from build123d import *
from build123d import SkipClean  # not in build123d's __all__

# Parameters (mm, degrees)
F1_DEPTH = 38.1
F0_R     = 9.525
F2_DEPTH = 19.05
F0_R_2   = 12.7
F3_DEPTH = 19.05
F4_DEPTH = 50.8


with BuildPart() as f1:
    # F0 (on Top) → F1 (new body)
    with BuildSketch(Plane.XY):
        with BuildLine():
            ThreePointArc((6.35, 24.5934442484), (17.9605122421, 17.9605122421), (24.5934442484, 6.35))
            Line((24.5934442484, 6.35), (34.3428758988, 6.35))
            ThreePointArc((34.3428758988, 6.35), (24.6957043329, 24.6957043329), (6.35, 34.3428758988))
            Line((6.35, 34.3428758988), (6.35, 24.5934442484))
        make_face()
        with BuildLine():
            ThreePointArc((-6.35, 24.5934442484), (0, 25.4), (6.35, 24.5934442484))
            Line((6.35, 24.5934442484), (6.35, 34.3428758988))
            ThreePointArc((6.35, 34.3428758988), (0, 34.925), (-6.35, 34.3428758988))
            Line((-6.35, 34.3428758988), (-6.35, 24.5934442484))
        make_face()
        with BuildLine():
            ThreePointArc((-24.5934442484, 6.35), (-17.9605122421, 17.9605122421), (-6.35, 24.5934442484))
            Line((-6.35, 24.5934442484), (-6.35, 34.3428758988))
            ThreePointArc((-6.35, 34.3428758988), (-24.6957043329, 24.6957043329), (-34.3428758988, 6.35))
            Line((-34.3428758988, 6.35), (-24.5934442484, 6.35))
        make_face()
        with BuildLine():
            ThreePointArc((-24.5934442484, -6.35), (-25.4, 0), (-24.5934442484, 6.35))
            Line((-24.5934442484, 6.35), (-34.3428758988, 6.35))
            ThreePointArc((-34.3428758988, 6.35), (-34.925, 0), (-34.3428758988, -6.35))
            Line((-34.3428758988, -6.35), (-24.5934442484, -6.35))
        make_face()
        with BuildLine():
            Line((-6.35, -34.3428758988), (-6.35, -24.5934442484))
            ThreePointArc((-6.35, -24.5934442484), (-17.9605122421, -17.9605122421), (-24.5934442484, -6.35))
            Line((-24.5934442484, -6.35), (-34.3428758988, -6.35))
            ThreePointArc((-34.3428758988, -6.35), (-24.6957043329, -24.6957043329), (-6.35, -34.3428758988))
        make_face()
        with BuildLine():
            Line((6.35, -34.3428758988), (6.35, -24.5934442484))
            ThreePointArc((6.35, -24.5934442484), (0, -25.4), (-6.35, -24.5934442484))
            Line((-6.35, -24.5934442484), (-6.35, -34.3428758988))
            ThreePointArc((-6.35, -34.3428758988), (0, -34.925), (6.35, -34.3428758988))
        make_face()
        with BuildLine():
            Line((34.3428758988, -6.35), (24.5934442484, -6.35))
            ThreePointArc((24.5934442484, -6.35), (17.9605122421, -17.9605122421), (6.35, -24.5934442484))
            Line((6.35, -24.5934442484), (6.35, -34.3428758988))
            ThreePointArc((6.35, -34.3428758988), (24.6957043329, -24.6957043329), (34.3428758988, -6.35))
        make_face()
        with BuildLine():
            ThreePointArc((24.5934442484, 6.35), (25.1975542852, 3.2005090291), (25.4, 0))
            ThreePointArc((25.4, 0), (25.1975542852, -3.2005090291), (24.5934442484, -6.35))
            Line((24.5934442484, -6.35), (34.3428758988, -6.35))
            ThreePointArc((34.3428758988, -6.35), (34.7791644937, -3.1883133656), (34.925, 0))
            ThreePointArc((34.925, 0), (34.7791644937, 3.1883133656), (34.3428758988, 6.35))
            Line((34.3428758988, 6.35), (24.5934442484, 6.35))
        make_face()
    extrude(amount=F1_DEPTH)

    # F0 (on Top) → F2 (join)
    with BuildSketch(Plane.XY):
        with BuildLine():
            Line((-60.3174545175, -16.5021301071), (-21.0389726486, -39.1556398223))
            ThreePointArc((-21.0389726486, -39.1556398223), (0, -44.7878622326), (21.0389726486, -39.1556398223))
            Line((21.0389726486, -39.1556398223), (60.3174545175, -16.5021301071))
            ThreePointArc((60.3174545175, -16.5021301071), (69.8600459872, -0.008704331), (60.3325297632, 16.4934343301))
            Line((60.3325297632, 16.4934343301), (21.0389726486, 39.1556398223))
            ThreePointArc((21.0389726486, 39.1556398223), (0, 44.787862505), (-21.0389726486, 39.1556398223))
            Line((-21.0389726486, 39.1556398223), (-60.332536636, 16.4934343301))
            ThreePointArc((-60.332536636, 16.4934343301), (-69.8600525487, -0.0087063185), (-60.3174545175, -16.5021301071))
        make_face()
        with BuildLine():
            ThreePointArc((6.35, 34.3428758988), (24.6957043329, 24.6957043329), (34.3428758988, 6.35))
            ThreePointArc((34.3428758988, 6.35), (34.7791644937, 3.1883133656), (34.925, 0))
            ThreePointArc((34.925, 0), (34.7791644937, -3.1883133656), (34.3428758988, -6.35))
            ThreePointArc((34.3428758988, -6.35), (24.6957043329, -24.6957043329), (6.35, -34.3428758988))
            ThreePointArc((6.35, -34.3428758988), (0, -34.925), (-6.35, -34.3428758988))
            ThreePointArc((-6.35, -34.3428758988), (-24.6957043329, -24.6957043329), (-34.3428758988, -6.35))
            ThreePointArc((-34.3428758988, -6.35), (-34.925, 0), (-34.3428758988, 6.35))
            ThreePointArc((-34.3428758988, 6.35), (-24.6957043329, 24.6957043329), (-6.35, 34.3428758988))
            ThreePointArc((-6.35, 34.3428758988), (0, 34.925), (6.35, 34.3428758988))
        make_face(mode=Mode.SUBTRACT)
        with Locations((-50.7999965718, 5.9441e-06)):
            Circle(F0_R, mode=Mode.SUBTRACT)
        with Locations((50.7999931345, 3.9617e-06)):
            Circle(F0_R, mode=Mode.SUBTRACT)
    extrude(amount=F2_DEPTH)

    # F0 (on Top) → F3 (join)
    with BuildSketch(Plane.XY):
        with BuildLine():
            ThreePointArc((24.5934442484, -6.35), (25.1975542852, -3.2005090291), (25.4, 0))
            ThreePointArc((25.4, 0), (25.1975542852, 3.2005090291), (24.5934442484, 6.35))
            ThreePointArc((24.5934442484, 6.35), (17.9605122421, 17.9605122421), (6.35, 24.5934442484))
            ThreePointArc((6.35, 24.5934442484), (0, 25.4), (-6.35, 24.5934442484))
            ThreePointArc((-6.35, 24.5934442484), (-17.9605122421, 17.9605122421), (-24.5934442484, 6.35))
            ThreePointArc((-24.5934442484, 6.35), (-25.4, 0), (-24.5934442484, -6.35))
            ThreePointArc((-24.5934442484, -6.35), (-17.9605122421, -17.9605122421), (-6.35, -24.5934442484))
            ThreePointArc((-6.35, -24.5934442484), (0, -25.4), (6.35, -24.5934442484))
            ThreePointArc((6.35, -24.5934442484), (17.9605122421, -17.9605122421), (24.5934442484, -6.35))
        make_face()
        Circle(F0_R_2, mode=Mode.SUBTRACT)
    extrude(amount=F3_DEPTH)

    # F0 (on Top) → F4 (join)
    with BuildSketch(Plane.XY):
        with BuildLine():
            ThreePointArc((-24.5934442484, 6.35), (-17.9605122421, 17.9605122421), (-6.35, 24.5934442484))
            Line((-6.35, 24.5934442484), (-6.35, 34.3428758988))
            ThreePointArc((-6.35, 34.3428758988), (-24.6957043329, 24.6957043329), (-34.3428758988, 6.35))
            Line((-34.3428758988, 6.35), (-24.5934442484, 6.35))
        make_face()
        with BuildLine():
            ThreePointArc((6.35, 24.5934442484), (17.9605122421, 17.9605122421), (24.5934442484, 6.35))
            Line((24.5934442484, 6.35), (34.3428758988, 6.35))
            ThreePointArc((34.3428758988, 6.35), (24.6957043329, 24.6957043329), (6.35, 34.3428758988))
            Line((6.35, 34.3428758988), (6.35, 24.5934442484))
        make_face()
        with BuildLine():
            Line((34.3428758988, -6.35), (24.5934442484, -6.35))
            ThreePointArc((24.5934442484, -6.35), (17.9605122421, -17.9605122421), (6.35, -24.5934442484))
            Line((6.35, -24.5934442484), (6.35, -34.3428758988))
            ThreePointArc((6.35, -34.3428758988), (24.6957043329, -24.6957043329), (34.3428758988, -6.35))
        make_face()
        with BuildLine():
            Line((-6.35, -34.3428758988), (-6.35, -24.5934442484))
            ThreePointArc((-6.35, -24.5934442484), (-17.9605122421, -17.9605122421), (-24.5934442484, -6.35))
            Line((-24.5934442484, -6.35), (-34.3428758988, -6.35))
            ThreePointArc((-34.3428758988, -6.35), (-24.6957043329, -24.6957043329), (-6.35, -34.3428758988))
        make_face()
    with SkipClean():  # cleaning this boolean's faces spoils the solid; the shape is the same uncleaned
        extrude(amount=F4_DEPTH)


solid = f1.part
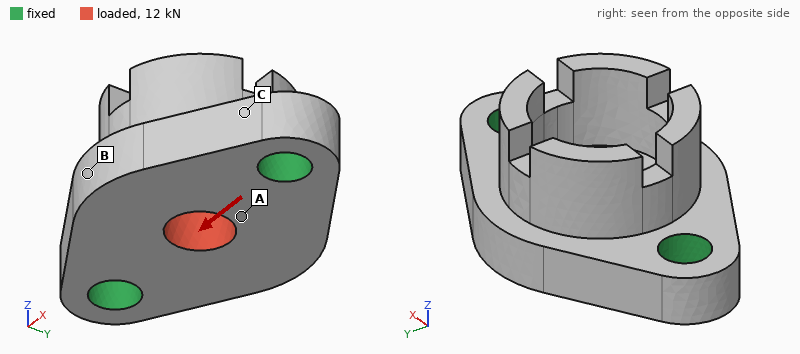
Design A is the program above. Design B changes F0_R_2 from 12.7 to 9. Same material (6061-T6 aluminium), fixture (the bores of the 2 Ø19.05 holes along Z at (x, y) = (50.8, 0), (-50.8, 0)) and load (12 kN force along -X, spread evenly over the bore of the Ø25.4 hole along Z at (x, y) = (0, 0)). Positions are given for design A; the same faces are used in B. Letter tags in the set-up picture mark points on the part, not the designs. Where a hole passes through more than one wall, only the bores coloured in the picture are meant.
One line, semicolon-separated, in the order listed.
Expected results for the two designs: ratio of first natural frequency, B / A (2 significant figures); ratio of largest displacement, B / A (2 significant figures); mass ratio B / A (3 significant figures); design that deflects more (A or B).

1.0; 1.1; 1.03; B
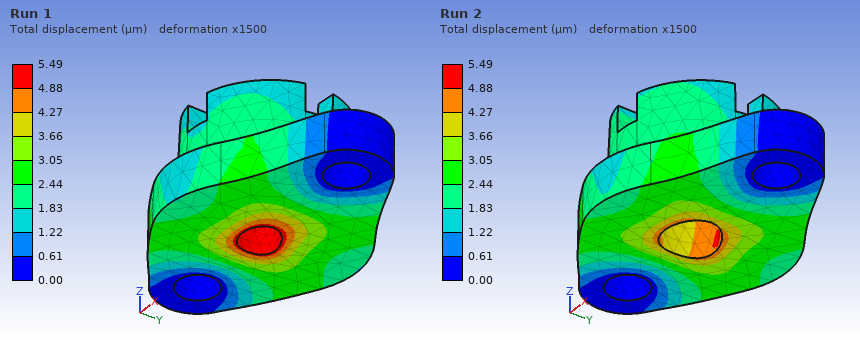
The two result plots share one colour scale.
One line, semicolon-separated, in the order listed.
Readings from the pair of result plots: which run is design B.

Run 1
